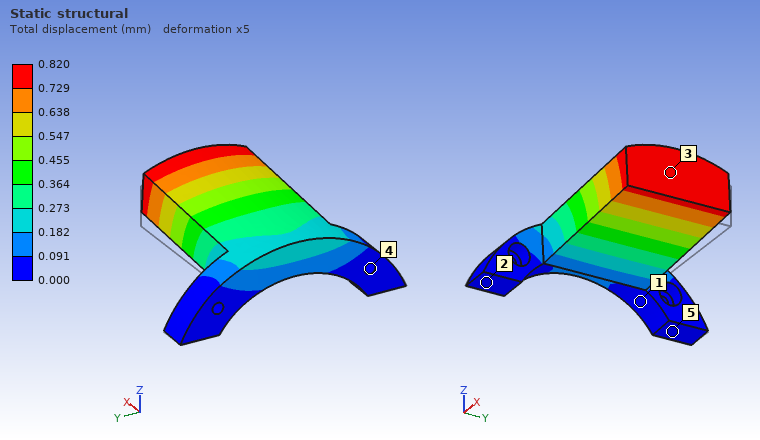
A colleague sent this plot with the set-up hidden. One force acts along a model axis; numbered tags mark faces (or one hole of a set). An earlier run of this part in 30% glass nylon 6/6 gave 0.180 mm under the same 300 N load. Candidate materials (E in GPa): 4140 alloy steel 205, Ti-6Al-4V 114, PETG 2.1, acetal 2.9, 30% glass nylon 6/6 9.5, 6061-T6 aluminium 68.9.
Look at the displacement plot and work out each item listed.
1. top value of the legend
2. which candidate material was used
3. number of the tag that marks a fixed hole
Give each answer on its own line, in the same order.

0.820 mm
PETG
4
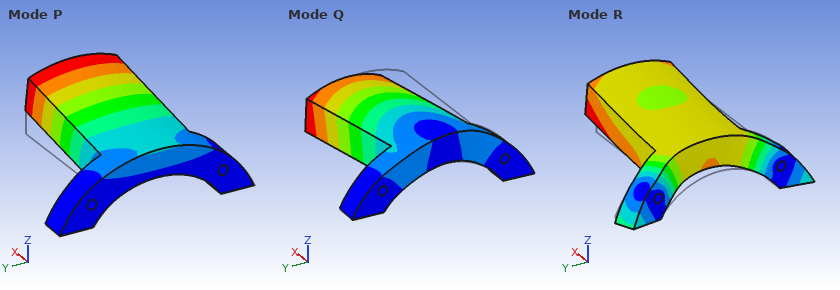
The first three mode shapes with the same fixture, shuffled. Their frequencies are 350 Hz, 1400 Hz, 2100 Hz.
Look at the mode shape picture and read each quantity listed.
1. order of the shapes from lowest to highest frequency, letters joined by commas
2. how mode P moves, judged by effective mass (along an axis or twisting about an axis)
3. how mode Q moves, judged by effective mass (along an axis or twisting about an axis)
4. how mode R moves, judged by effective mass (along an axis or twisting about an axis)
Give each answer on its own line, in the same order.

P, Q, R
along Z
along Y
along X
